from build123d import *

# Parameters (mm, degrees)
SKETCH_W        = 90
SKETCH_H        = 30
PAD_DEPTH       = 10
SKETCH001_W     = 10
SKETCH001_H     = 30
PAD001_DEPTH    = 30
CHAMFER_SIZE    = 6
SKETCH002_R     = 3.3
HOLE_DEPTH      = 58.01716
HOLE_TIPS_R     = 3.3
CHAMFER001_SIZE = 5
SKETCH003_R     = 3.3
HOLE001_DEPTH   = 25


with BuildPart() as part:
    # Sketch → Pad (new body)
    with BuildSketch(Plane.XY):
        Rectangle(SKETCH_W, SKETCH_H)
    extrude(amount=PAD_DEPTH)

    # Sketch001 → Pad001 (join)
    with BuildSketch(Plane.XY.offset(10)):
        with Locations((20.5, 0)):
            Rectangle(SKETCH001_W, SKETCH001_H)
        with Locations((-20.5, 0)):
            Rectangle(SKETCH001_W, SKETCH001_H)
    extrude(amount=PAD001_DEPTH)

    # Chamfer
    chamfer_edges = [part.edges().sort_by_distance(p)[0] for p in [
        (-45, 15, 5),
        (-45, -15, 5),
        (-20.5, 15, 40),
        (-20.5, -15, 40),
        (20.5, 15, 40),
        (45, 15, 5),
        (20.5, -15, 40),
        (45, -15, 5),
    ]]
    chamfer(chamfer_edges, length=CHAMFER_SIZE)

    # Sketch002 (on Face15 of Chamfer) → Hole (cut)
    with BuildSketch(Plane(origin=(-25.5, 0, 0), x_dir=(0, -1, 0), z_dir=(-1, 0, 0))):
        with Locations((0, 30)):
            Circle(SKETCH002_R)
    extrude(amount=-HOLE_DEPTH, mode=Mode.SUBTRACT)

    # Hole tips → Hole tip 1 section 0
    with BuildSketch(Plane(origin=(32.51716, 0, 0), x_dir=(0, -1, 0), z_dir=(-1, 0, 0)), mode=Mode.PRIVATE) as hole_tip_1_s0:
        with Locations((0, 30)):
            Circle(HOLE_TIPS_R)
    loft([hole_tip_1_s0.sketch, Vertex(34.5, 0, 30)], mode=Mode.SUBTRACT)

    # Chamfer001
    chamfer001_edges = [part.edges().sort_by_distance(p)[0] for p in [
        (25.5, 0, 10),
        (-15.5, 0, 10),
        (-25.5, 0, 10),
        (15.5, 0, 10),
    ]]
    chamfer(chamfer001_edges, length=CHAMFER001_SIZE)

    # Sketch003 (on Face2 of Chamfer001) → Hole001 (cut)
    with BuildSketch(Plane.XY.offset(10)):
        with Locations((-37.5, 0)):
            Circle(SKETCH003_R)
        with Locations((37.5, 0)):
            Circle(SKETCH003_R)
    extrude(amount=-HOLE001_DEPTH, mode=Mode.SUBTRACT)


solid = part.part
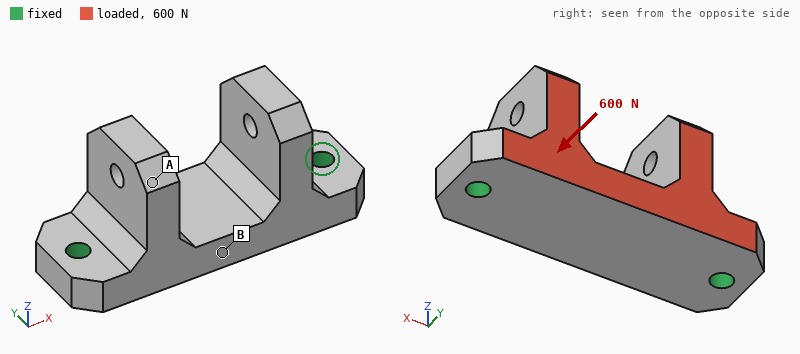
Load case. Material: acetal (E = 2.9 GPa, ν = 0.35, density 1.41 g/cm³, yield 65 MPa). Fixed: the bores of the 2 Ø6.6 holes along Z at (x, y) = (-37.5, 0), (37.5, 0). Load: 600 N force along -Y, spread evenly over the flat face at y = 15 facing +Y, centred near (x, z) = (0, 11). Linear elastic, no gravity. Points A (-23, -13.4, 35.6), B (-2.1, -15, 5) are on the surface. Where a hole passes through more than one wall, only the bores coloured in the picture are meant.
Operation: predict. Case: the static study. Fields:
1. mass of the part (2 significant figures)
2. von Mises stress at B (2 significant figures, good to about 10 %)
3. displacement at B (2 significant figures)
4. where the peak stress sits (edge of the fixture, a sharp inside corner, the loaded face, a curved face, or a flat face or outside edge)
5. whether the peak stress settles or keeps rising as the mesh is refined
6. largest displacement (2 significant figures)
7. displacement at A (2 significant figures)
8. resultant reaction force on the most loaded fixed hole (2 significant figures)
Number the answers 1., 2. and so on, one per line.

1. 62 g
2. 2.3 MPa
3. 0.052 mm
4. edge of the fixture
5. keeps rising
6. 0.13 mm
7. 0.11 mm
8. 300 N
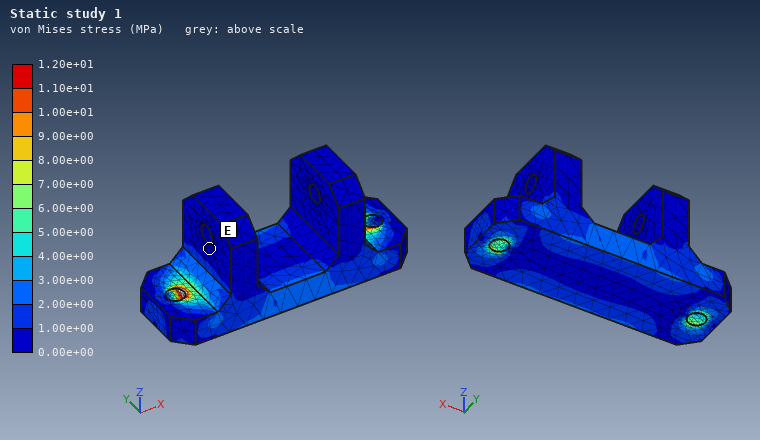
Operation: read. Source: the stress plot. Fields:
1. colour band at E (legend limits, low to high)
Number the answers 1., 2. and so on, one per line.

1. 0.00e+00 to 1.00e+00 MPa
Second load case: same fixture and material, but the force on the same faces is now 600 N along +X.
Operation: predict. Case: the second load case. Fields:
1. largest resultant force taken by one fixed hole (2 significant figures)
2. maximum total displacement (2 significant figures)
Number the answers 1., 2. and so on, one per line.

1. 320 N
2. 69 µm
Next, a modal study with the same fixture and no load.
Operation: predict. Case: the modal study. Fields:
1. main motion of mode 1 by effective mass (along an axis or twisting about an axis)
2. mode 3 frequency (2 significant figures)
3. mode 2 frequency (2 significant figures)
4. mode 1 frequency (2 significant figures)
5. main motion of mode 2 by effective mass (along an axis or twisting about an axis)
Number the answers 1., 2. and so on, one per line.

1. along Z
2. 2200 Hz
3. 1500 Hz
4. 1400 Hz
5. along Y
